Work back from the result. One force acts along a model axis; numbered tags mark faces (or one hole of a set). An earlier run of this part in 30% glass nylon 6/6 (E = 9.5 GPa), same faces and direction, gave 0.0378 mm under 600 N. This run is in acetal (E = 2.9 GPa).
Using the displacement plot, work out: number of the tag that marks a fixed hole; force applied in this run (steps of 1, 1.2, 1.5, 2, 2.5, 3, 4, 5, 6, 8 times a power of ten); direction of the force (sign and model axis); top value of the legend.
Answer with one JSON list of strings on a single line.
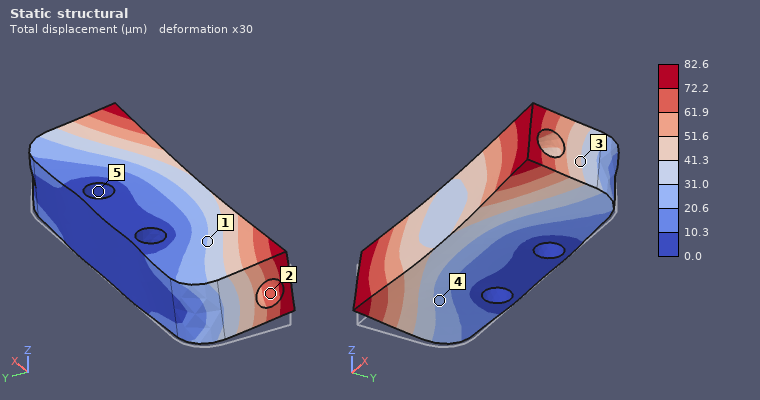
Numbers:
["5", "400 N", "+Z", "82.6 µm"]
